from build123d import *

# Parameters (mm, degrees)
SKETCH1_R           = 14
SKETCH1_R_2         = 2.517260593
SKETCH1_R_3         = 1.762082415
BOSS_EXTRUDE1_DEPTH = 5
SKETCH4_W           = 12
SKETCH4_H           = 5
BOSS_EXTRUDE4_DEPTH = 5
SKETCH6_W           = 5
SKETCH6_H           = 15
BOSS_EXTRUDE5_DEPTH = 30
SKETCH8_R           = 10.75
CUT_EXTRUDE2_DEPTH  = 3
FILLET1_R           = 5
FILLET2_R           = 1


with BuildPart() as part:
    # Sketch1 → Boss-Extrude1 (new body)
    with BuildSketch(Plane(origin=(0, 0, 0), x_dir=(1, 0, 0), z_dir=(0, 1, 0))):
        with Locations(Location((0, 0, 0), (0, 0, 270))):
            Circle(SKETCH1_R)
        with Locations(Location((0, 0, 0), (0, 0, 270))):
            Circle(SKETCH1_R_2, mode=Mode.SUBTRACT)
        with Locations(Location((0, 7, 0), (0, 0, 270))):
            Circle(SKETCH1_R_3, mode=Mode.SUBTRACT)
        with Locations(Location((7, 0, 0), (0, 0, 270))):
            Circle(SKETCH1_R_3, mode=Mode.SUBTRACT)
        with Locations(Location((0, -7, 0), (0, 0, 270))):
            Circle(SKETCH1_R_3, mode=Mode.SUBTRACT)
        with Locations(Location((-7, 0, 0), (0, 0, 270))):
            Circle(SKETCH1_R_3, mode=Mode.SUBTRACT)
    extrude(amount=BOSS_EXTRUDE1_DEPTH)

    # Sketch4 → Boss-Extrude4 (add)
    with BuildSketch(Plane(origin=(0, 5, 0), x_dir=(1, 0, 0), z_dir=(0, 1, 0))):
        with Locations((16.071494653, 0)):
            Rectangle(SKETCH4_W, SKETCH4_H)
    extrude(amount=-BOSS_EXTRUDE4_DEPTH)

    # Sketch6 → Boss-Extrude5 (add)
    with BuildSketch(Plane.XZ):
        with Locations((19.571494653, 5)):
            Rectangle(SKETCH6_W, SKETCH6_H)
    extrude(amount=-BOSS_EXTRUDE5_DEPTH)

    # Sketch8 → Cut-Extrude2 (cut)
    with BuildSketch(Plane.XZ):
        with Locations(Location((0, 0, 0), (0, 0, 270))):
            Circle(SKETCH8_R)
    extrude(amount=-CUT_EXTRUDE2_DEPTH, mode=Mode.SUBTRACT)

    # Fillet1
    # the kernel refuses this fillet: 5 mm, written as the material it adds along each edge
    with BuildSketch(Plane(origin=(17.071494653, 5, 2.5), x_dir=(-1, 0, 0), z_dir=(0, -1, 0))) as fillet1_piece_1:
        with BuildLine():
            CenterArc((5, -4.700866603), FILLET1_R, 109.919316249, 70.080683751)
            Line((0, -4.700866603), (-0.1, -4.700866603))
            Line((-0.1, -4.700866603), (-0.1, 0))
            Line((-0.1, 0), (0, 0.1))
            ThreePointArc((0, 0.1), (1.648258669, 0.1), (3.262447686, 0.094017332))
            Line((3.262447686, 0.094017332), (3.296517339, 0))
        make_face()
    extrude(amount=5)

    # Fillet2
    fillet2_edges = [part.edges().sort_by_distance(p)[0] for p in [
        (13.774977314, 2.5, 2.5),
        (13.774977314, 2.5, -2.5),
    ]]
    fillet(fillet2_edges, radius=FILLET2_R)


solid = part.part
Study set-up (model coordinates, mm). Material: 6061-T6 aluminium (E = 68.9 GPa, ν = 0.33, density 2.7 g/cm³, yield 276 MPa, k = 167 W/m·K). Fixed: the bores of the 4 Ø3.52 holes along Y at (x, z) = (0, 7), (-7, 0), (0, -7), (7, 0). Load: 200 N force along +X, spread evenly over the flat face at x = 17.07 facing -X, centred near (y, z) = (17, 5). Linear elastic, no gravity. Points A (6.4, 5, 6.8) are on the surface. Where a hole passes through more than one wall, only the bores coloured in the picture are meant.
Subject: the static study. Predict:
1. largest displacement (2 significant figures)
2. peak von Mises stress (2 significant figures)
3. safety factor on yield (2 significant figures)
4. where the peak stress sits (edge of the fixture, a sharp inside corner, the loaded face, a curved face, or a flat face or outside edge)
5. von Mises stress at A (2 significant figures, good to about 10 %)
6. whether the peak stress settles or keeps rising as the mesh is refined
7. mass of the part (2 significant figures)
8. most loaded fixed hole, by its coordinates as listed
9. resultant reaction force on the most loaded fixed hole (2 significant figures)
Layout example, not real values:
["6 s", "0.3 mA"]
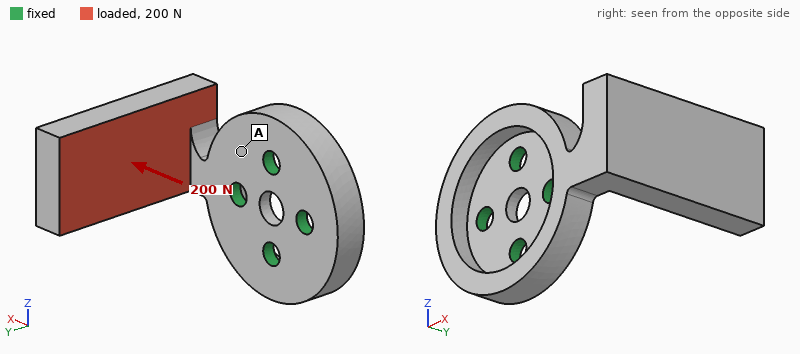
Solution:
["0.37 mm", "330 MPa", "0.83", "a curved face", "30 MPa", "settles", "11 g", "(7, 0)", "410 N"]
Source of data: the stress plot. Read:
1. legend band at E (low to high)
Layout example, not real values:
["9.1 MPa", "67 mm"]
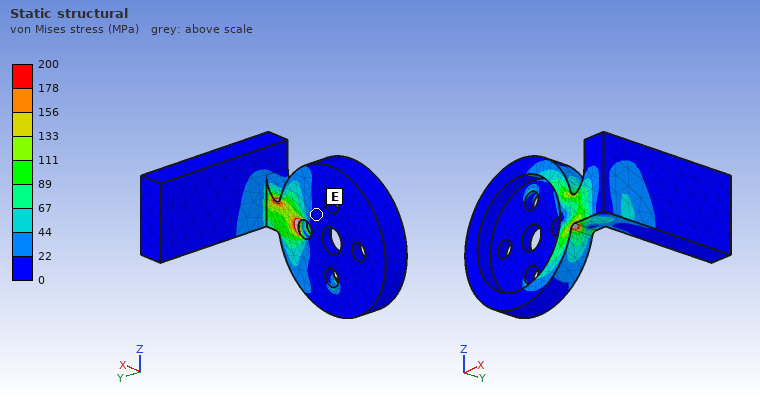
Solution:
["0 to 22 MPa"]
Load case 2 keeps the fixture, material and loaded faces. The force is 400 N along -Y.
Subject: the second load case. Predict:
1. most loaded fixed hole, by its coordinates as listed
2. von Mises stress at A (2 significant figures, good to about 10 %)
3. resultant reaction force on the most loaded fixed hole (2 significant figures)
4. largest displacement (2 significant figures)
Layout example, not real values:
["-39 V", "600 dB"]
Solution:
["(7, 0)", "47 MPa", "630 N", "0.31 mm"]
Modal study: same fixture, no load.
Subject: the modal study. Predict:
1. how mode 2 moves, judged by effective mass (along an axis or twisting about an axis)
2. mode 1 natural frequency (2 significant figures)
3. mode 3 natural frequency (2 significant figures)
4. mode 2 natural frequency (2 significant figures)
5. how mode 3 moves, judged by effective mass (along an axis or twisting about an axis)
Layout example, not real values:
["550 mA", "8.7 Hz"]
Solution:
["along Z", "1800 Hz", "7000 Hz", "2300 Hz", "along Y"]
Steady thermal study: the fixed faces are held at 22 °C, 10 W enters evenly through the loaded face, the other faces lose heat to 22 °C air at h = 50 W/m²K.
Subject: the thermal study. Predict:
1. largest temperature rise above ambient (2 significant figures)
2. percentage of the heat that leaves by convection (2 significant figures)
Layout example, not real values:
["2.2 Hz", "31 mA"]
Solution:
["29 K", "13 %"]
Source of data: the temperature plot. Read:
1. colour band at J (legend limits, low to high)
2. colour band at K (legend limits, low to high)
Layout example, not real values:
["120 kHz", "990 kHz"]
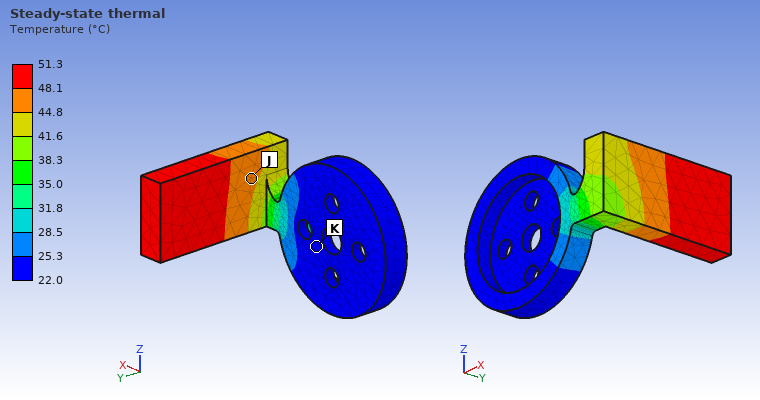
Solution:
["44.8 to 48.1 °C", "22.0 to 25.3 °C"]
